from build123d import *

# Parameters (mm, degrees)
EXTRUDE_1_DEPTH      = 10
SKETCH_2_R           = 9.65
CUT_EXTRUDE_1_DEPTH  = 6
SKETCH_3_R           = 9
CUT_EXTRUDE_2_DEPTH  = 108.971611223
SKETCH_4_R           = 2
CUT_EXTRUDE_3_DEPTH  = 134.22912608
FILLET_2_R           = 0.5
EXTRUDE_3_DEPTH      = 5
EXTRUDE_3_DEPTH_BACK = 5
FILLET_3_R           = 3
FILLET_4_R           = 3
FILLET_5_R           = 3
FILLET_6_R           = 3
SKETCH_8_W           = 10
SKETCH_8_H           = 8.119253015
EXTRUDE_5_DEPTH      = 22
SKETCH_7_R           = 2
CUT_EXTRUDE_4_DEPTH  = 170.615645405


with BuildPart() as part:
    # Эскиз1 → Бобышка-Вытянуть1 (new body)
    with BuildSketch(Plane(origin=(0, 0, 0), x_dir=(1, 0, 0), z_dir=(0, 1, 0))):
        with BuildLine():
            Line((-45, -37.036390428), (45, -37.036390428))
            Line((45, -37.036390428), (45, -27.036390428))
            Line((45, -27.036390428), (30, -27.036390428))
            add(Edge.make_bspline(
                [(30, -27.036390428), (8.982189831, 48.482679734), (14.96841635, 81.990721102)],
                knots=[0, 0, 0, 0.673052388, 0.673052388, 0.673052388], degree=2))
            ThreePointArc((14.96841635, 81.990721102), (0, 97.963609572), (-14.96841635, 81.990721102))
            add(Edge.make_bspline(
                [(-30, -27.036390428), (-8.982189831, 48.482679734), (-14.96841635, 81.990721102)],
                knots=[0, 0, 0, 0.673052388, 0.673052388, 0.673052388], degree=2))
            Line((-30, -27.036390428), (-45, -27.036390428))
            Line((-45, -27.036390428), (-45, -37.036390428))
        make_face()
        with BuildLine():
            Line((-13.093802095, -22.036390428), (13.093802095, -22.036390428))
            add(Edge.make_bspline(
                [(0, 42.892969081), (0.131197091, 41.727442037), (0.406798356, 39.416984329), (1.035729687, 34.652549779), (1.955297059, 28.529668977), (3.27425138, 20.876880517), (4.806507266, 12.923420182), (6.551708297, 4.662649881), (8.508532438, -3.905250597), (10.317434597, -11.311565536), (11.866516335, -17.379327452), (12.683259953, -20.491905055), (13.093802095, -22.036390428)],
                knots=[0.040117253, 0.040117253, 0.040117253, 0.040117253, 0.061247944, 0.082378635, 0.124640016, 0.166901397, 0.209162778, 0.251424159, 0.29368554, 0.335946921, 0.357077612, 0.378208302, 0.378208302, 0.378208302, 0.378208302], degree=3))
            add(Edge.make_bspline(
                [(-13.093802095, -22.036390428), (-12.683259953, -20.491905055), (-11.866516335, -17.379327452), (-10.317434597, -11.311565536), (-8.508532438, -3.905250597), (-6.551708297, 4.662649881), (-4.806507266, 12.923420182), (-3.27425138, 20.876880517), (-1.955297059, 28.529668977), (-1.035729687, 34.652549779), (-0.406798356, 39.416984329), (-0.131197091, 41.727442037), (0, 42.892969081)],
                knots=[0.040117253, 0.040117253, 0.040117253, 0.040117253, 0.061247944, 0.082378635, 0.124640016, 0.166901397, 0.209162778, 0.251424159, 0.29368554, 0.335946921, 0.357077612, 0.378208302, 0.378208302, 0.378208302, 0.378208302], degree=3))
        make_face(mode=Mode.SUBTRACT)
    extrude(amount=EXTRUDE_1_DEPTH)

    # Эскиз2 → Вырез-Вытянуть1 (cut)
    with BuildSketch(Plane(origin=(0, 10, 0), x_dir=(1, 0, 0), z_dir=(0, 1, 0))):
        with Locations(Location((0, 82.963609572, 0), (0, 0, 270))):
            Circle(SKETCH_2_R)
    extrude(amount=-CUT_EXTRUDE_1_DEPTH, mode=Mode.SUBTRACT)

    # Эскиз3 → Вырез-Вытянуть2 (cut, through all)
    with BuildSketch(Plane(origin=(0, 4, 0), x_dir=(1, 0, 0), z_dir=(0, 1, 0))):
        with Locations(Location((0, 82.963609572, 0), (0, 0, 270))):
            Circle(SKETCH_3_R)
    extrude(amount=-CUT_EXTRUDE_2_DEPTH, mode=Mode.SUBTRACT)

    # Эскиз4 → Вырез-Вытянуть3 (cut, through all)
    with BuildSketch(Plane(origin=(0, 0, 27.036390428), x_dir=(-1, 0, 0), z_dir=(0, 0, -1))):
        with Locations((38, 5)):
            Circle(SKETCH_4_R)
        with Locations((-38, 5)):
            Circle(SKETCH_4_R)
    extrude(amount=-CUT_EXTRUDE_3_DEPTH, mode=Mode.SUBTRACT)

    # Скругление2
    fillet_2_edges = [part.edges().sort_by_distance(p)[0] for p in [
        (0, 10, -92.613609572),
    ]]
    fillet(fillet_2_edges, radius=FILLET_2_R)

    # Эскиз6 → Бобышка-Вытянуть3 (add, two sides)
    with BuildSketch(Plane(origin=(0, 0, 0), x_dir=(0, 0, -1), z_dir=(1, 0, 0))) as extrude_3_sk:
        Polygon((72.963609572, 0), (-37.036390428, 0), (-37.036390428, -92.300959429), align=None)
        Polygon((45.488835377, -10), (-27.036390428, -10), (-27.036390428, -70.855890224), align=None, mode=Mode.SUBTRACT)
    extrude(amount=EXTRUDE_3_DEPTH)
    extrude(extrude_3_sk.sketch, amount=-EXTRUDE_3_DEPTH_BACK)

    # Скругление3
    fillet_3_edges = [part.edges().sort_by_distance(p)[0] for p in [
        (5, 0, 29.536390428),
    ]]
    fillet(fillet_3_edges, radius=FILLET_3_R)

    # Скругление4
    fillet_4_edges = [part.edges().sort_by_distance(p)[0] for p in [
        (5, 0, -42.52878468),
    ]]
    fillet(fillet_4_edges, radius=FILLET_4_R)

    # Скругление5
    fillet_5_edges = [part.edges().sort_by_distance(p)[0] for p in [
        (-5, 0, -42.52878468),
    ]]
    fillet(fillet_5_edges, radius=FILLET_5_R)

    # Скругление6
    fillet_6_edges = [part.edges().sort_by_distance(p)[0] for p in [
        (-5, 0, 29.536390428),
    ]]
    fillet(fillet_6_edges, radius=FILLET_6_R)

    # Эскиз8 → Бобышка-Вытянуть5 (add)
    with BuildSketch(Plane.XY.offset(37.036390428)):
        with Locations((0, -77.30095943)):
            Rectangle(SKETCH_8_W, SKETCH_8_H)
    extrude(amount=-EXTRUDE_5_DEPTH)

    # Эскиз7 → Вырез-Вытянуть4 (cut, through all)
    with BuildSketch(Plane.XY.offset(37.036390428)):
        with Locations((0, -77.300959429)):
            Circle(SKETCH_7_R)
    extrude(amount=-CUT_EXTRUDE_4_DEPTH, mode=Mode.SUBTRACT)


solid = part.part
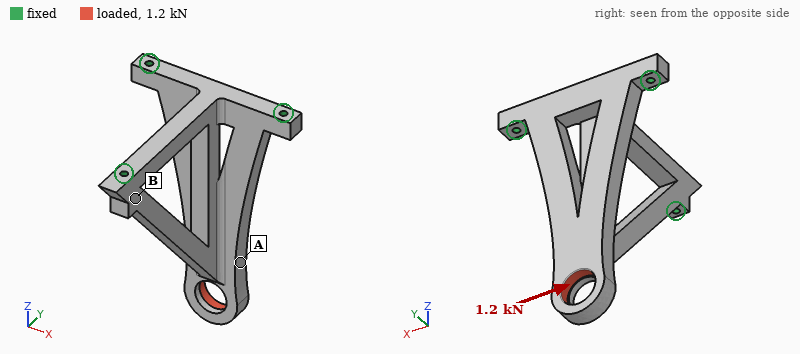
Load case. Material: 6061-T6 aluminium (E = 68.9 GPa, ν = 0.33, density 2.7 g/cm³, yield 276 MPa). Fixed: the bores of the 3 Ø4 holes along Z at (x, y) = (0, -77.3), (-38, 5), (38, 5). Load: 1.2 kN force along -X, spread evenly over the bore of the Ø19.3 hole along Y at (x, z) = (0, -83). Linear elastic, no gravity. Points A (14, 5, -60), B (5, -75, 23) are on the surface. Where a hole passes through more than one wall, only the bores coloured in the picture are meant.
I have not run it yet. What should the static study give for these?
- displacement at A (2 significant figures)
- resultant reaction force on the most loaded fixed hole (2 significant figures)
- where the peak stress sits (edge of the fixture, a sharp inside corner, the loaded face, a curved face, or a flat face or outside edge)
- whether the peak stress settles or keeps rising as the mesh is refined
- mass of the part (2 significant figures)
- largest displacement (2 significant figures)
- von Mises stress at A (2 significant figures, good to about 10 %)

0.14 mm
2.2 kN
edge of the fixture
keeps rising
200 g
0.26 mm
23 MPa
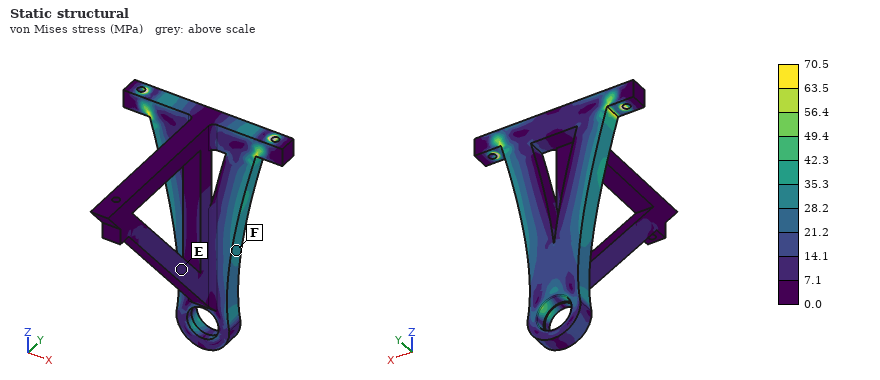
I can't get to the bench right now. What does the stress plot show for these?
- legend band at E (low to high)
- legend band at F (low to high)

7.1 to 14.1 MPa
28.2 to 35.3 MPa
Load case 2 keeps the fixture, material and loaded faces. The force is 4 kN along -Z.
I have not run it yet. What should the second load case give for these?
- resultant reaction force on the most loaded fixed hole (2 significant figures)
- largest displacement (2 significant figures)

2.2 kN
0.14 mm
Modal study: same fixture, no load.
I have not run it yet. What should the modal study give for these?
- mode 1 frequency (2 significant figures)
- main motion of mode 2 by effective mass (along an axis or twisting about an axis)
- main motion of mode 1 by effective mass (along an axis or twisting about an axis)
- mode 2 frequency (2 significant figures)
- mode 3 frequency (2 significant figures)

2200 Hz
along Y
along X
2700 Hz
3200 Hz
